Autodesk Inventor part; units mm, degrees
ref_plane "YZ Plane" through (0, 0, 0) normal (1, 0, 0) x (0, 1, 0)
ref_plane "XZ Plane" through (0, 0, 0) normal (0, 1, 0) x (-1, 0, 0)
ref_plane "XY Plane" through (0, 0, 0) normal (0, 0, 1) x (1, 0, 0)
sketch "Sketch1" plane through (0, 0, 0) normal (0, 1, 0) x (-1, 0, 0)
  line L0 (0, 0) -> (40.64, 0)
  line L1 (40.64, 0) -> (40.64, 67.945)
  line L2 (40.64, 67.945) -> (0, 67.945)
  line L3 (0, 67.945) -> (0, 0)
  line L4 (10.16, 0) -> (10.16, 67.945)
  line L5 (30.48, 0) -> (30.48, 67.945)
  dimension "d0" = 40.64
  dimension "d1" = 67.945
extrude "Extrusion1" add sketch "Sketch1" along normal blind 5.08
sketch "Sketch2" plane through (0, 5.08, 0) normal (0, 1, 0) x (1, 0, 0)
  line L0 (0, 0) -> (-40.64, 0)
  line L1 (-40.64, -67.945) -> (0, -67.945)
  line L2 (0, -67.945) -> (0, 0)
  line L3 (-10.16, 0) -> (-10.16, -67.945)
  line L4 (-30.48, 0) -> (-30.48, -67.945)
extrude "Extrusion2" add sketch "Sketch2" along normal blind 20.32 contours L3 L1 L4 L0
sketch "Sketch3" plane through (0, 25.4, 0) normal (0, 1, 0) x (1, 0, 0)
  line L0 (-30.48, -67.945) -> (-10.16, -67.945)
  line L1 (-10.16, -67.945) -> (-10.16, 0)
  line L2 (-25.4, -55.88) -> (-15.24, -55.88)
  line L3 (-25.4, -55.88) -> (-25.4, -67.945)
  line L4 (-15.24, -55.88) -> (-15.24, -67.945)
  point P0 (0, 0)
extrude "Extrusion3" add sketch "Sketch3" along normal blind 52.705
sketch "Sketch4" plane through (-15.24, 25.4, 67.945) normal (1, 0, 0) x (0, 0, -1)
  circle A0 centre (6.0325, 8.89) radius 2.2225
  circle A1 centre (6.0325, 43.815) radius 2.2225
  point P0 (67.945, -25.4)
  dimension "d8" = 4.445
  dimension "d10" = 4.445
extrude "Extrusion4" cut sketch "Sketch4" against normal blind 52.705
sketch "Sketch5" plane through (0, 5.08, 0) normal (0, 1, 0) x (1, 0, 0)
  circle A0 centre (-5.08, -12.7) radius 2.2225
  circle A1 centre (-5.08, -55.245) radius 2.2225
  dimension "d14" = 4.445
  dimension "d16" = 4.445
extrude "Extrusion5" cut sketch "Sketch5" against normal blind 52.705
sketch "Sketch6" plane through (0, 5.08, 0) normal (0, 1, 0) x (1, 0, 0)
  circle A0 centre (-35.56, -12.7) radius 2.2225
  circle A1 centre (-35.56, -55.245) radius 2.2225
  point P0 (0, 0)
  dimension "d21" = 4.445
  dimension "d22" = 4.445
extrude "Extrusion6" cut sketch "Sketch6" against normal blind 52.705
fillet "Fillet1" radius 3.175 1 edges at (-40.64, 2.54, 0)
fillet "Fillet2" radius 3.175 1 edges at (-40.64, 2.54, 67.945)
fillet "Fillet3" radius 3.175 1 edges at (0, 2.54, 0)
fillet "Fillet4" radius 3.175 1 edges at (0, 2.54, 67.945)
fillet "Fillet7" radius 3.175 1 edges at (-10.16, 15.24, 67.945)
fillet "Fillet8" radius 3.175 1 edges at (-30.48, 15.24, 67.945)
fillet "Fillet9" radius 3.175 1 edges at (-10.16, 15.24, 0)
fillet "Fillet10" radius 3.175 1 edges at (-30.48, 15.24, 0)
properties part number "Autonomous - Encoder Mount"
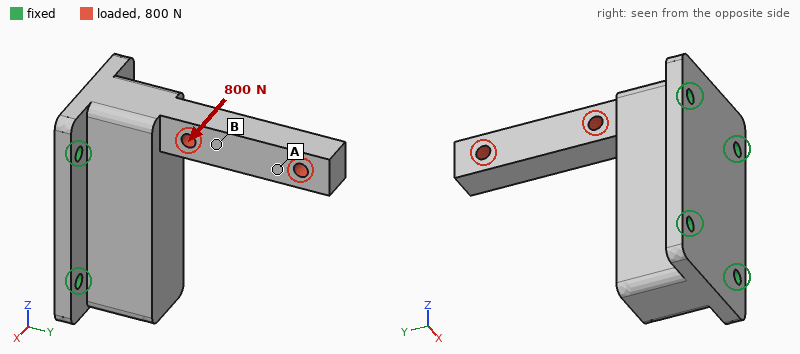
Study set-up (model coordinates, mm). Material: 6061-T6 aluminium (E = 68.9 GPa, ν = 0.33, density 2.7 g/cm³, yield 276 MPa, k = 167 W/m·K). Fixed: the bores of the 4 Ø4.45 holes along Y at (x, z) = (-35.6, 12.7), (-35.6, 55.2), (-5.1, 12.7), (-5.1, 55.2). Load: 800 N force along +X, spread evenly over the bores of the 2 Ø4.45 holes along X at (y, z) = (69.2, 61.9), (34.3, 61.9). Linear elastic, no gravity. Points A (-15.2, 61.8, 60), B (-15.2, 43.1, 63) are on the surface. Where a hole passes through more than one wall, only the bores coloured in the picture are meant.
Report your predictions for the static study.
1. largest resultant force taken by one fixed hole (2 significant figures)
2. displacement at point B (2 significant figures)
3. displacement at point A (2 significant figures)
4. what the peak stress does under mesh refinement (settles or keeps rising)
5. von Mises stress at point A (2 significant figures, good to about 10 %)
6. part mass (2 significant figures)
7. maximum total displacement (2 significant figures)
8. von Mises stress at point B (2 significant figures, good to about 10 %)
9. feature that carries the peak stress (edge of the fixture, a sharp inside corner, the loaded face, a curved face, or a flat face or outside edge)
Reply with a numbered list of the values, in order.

1. 1.2 kN
2. 0.10 mm
3. 0.24 mm
4. keeps rising
5. 14 MPa
6. 130 g
7. 0.37 mm
8. 47 MPa
9. a sharp inside corner
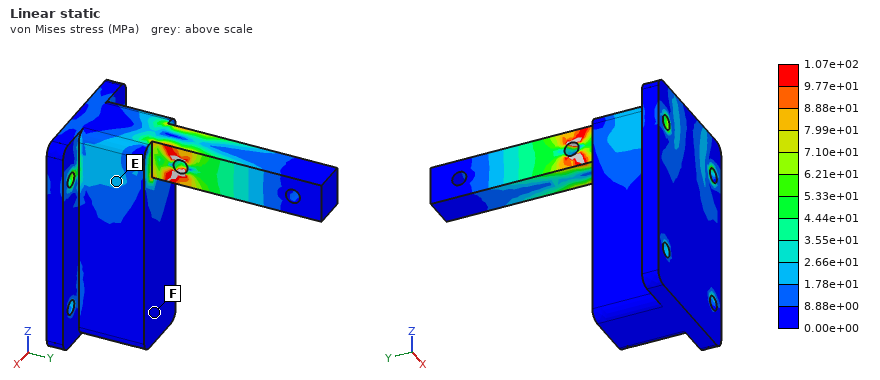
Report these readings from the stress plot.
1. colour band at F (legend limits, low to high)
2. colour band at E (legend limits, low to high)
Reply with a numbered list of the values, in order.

1. 0.00e+00 to 8.88e+00 MPa
2. 1.78e+01 to 2.66e+01 MPa
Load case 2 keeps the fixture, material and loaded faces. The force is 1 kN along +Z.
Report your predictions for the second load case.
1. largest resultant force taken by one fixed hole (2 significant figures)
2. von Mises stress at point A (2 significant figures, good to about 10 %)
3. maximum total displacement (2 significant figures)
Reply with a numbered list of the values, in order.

1. 750 N
2. 12 MPa
3. 0.31 mm
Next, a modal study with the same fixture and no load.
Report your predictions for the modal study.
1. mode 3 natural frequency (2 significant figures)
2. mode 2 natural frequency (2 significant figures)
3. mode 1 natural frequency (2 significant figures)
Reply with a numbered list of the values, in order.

1. 9400 Hz
2. 2800 Hz
3. 2300 Hz
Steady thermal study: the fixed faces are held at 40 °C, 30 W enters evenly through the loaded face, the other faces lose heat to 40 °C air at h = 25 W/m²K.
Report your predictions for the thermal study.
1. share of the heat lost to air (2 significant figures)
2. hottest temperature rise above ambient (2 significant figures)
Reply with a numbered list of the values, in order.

1. 11 %
2. 54 K
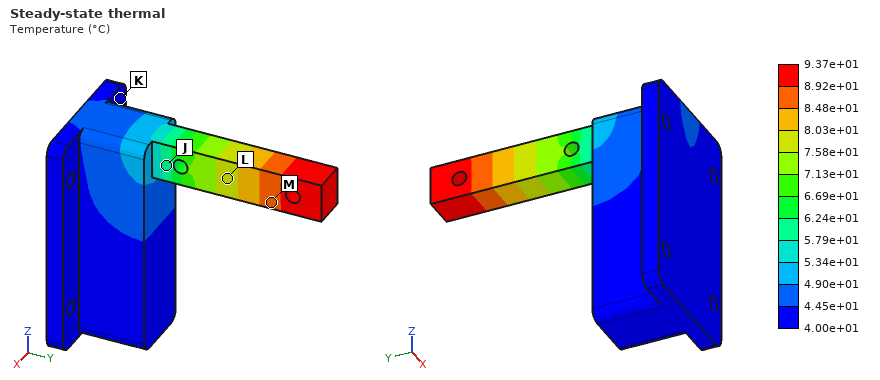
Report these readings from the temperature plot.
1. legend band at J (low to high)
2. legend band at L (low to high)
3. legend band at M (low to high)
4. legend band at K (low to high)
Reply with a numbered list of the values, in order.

1. 5.79e+01 to 6.24e+01 °C
2. 7.58e+01 to 8.03e+01 °C
3. 8.48e+01 to 8.92e+01 °C
4. 4.00e+01 to 4.45e+01 °C
